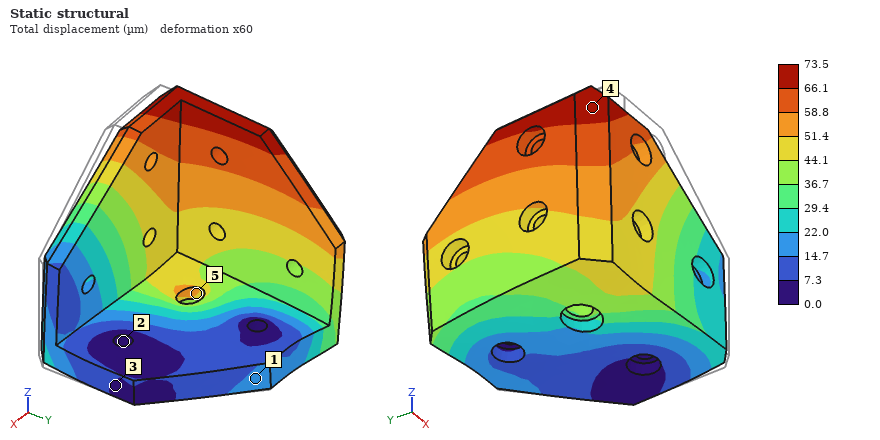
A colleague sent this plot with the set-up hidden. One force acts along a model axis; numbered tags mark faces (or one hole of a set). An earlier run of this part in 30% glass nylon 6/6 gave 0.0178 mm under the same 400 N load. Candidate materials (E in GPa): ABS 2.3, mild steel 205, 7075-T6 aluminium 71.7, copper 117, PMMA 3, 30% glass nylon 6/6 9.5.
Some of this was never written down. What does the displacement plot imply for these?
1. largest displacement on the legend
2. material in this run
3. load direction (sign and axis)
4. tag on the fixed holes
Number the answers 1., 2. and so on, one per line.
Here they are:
1. 73.5 µm
2. ABS
3. +Y
4. 2
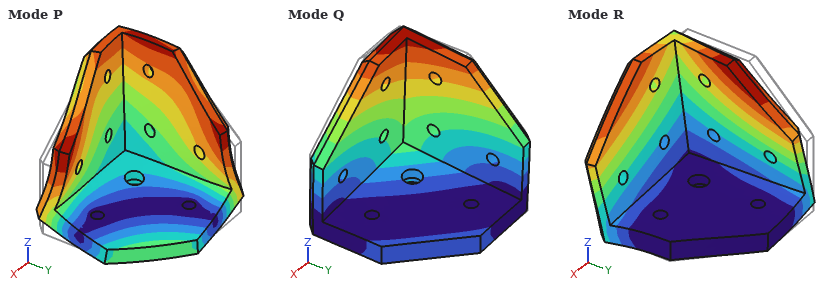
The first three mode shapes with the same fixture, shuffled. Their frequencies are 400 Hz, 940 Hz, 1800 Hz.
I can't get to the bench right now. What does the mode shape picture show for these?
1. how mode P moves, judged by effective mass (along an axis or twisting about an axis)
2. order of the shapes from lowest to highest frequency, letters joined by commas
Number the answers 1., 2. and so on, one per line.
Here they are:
1. along Z
2. Q, R, P
